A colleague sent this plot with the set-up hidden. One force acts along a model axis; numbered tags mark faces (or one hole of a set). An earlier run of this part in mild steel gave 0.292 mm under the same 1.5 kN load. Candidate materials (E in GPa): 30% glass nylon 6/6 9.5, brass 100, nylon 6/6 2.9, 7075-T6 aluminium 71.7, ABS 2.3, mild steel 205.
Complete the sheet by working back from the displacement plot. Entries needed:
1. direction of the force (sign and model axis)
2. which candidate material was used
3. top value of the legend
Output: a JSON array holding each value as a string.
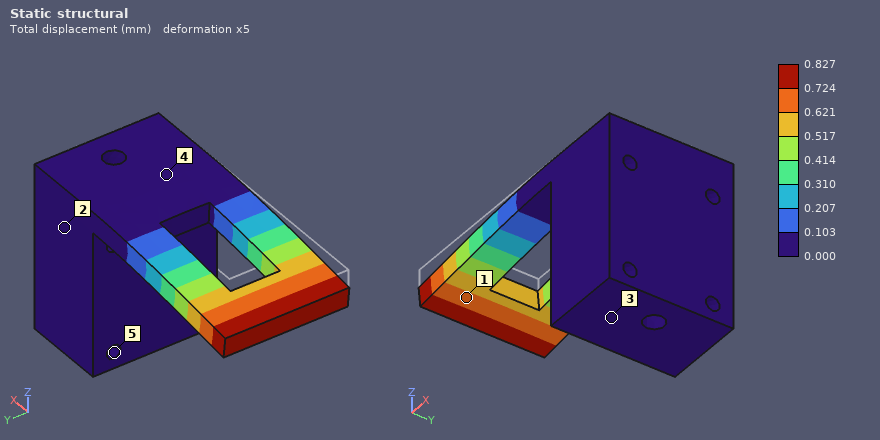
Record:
["-Z", "7075-T6 aluminium", "0.827 mm"]
